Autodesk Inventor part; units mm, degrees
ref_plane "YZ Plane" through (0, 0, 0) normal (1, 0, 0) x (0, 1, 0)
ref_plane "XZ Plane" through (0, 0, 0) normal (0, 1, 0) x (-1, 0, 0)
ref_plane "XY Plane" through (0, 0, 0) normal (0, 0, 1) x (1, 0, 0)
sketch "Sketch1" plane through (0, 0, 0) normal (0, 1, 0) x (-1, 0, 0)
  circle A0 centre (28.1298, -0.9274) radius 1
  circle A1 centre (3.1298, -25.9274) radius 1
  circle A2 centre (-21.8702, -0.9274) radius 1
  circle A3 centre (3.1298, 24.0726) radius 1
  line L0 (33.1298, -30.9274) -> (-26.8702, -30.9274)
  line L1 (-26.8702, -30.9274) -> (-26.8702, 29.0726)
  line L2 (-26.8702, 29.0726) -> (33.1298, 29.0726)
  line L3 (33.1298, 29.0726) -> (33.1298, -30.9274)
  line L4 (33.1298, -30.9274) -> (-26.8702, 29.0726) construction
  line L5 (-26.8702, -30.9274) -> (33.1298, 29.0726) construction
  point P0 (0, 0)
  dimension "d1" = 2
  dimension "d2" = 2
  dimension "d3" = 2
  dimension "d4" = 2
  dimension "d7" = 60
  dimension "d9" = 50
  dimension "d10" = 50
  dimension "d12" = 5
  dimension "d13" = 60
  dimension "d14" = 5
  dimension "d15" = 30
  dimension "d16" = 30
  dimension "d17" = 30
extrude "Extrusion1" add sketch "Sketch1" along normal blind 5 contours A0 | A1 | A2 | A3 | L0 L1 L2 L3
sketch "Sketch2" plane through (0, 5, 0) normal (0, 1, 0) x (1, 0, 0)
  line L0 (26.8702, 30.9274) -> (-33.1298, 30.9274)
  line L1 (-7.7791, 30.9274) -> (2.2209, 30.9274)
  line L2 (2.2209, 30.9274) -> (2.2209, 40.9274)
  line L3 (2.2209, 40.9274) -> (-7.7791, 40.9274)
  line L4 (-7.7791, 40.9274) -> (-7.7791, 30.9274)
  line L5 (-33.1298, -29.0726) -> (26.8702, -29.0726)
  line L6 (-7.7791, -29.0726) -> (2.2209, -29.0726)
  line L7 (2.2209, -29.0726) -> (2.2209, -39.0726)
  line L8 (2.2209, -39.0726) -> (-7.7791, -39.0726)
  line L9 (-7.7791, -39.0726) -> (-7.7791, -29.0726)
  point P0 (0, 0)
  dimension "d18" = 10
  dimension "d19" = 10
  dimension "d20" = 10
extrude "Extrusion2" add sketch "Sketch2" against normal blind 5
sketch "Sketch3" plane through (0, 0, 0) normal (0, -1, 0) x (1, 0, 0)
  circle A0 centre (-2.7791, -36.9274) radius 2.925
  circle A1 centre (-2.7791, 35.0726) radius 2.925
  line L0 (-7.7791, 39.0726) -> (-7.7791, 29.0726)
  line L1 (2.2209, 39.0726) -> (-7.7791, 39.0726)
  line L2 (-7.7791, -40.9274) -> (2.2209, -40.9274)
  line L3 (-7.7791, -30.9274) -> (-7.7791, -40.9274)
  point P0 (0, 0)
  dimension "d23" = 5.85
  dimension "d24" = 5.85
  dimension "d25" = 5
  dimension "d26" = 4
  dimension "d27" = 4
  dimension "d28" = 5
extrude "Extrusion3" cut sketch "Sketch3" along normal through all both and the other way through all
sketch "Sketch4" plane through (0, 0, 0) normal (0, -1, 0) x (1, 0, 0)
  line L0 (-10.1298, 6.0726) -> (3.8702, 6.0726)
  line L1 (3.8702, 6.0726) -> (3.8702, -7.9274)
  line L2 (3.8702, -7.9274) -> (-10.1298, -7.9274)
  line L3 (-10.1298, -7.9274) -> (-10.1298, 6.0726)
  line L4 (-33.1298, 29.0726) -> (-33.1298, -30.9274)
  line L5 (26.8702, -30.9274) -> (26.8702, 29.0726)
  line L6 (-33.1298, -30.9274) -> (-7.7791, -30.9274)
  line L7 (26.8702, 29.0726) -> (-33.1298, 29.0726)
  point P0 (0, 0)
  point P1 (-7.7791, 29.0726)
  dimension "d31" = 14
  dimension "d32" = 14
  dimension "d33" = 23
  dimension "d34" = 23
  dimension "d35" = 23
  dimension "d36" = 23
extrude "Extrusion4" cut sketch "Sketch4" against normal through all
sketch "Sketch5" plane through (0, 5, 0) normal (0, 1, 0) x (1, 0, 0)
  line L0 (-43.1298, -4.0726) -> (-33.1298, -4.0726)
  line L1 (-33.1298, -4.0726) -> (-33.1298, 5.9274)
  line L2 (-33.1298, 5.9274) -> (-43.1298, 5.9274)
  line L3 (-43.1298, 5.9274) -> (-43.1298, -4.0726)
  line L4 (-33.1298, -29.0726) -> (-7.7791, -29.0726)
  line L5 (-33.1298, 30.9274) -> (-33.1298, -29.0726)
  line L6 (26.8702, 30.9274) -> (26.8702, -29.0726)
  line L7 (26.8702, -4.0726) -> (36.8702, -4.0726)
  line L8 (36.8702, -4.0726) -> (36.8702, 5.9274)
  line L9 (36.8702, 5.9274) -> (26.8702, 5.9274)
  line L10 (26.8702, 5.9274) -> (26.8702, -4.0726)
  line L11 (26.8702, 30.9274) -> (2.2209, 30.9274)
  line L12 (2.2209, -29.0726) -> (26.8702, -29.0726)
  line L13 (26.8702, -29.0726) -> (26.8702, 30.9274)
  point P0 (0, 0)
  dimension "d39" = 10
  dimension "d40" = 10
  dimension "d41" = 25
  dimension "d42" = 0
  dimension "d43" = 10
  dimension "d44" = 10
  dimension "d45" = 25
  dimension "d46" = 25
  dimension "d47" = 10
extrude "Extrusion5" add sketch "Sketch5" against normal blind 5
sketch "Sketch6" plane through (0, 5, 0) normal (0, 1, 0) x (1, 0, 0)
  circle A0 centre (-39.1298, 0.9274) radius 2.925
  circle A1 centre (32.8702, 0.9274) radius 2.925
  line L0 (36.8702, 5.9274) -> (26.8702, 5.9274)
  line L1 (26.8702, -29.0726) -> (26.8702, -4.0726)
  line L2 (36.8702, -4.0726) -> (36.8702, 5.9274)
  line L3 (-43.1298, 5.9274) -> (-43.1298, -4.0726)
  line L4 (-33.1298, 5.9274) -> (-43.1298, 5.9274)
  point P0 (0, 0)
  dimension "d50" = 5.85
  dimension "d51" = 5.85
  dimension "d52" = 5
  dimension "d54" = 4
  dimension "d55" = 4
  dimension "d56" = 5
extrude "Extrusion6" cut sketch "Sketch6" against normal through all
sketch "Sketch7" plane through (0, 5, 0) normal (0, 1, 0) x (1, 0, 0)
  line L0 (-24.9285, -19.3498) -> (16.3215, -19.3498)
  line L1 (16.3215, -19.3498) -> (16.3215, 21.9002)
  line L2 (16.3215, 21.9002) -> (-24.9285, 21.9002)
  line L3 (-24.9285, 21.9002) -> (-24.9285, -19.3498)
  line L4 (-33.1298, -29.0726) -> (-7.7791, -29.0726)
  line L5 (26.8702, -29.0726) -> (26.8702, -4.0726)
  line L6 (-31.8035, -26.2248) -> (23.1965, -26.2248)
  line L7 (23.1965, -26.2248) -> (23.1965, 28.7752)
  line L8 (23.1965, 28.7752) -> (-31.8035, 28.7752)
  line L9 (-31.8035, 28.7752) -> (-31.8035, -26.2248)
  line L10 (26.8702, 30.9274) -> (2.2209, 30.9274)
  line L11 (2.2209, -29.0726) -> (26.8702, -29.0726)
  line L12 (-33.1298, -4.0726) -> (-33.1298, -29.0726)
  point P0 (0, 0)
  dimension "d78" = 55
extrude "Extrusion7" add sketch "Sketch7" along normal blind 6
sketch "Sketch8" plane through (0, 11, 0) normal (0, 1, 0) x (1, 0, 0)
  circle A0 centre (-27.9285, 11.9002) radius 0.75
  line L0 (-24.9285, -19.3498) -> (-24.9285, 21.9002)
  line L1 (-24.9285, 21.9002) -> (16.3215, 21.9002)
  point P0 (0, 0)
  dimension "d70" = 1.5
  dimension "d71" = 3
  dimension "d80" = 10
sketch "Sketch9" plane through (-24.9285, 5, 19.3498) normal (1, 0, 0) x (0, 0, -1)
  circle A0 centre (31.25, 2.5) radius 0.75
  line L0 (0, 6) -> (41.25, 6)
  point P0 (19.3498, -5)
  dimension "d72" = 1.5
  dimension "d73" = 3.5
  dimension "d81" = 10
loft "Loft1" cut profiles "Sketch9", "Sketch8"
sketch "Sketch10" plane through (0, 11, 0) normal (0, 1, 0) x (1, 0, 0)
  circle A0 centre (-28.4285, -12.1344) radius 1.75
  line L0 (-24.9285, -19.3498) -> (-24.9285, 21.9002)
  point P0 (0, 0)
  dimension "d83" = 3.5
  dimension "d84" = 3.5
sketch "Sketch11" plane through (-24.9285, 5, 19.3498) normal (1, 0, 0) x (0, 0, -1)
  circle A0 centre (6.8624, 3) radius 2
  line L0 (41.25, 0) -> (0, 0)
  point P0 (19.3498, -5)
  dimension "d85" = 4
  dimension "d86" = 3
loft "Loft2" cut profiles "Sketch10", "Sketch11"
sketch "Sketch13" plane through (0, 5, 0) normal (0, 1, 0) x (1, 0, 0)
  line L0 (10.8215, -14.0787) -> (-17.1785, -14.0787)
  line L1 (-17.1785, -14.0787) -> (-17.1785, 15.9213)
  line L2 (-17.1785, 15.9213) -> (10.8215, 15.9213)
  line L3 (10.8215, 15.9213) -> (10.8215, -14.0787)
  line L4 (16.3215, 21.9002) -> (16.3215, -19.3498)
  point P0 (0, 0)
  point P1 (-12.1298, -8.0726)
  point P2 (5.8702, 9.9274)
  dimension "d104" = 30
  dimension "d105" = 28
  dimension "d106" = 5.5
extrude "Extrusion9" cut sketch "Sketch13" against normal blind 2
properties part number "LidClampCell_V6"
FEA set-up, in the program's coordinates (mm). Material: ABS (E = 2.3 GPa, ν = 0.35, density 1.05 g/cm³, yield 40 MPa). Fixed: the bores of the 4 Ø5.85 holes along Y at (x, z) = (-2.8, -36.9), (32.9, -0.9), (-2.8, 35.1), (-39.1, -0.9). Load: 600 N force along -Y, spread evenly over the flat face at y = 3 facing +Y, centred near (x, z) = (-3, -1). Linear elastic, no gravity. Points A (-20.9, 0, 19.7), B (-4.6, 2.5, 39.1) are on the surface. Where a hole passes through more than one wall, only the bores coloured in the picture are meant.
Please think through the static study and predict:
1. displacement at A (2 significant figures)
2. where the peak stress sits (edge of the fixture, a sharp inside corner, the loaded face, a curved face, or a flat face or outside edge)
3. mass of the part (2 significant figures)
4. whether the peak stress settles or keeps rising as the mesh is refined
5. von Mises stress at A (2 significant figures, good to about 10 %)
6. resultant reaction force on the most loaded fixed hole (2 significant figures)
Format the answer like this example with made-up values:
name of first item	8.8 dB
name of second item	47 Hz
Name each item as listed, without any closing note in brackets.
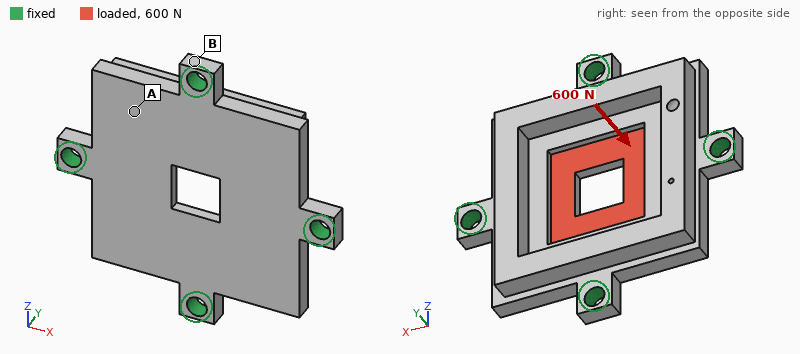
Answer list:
displacement at A	0.15 mm
where the peak stress sits	edge of the fixture
mass of the part	26 g
whether the peak stress settles or keeps rising as the mesh is refined	keeps rising
von Mises stress at A	6.1 MPa
resultant reaction force on the most loaded fixed hole	150 N
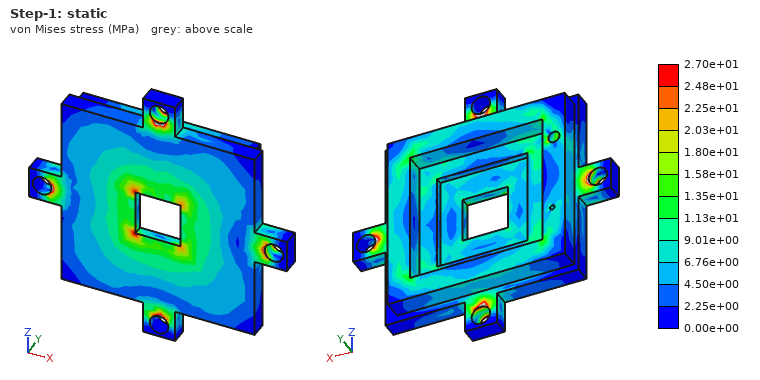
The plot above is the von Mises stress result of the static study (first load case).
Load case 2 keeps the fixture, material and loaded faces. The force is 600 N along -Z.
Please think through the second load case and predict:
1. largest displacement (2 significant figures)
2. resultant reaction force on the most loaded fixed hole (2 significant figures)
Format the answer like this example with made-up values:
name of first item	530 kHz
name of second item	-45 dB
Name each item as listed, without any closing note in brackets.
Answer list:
largest displacement	42 µm
resultant reaction force on the most loaded fixed hole	220 N
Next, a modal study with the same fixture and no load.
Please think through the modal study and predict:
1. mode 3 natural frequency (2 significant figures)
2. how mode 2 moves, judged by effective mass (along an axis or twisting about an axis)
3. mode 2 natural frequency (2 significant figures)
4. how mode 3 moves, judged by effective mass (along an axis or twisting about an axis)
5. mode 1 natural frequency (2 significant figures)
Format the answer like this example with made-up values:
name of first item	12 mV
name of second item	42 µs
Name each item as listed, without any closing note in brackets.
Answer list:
mode 3 natural frequency	2500 Hz
how mode 2 moves, judged by effective mass	along Y
mode 2 natural frequency	2300 Hz
how mode 3 moves, judged by effective mass	twisting about Z
mode 1 natural frequency	1800 Hz
